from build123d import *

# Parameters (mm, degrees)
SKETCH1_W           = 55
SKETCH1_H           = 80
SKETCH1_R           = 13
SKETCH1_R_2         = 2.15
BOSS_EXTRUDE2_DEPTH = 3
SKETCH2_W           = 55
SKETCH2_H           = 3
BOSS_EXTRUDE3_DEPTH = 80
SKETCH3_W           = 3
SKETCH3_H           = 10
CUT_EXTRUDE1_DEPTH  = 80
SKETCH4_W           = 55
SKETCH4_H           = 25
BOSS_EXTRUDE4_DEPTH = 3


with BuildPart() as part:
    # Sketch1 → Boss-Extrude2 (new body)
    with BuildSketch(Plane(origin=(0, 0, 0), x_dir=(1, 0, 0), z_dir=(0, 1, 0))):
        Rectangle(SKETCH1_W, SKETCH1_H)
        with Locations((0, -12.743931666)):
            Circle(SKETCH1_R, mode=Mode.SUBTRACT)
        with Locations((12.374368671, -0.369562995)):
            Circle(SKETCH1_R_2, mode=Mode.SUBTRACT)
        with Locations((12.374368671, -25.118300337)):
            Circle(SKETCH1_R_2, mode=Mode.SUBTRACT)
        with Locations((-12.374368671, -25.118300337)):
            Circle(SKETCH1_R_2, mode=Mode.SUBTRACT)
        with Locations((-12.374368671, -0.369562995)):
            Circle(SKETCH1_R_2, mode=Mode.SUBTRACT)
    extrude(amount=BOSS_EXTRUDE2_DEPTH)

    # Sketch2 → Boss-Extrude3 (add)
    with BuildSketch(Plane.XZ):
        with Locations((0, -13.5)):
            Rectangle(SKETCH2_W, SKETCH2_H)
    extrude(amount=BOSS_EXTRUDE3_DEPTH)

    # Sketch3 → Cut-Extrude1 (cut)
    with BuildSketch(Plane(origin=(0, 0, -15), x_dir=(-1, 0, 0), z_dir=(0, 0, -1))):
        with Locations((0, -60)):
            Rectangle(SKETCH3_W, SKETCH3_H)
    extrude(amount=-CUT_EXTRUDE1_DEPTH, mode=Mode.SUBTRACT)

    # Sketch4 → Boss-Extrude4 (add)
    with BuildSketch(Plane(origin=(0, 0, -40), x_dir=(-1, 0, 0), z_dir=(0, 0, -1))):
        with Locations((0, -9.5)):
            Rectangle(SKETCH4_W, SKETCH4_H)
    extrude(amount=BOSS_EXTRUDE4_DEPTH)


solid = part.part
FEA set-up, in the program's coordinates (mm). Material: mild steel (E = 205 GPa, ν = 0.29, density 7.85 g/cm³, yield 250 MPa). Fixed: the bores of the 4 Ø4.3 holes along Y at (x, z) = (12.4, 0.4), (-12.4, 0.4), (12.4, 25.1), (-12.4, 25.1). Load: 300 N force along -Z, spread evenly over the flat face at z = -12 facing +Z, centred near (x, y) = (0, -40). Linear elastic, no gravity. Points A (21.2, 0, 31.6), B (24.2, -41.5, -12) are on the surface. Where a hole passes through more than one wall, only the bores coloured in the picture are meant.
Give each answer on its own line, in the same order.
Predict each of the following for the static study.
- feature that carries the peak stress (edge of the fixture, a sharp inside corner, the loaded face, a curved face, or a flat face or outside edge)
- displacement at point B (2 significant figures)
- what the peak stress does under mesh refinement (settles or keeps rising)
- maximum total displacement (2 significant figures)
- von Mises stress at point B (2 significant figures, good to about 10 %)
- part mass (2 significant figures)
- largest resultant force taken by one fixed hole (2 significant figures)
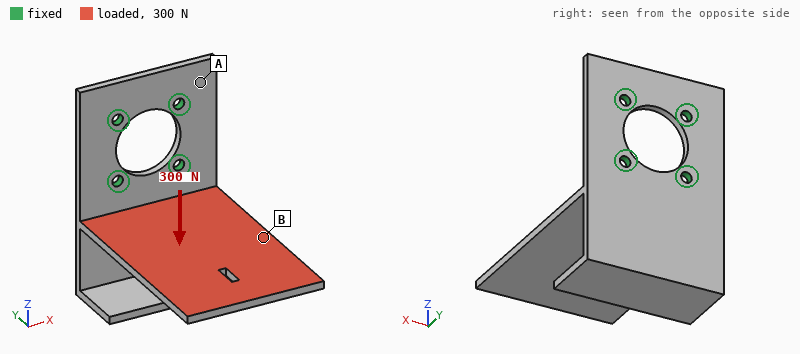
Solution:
edge of the fixture
0.57 mm
keeps rising
1.3 mm
35 MPa
230 g
150 N
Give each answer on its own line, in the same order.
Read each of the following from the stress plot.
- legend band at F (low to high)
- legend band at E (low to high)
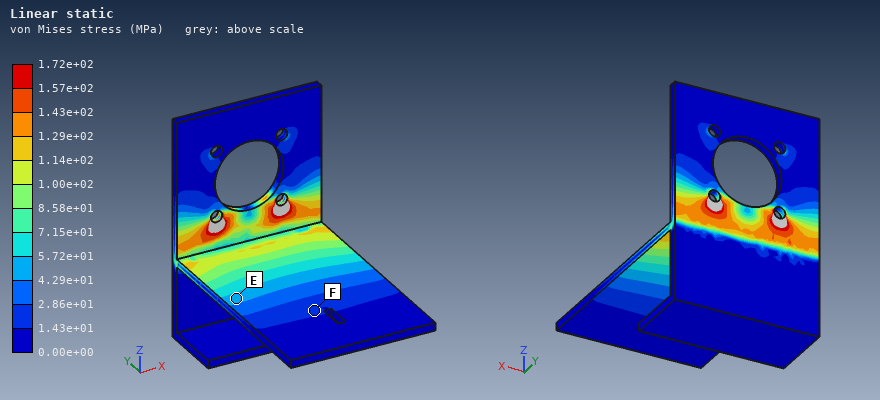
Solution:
1.43e+01 to 2.86e+01 MPa
4.29e+01 to 5.72e+01 MPa
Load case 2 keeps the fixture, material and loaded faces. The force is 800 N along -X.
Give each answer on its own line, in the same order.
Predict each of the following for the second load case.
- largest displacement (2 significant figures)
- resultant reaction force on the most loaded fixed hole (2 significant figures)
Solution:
0.26 mm
1.2 kN
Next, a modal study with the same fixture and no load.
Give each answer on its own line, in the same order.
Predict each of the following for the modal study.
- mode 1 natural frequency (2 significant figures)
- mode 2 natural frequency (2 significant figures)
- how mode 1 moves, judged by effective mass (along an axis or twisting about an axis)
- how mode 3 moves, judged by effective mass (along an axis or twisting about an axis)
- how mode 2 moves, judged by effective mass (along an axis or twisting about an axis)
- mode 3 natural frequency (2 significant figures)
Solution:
290 Hz
860 Hz
along Z
along X
along Y
930 Hz
